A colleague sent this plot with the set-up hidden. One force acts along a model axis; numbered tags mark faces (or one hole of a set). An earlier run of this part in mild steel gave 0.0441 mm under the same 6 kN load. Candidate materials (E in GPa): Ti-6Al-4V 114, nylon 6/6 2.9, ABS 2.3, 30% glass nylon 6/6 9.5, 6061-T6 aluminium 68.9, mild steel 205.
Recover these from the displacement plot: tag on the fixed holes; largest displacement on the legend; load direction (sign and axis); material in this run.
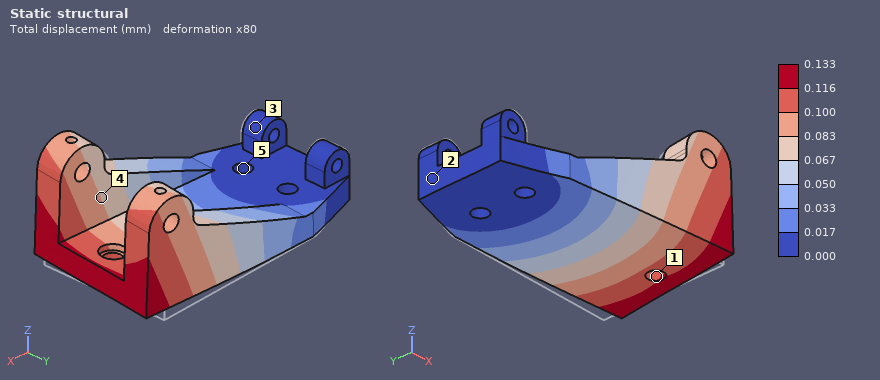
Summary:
5
0.133 mm
-Y
6061-T6 aluminium
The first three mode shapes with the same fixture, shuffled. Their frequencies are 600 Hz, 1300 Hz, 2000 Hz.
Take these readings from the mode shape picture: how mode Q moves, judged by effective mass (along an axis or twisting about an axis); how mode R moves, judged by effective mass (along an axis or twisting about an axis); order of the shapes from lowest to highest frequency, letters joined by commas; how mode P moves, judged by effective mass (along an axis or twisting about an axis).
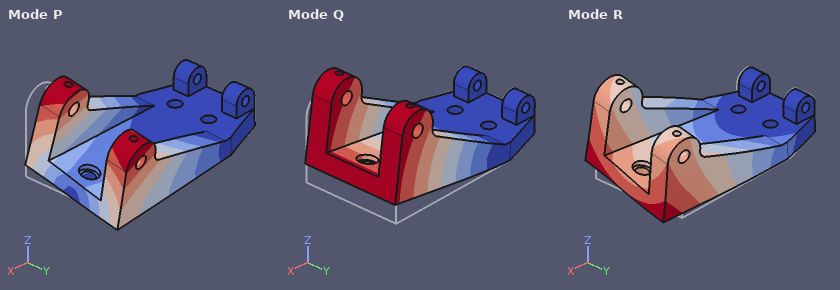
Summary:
along Z
along Y
Q, P, R
along Y
